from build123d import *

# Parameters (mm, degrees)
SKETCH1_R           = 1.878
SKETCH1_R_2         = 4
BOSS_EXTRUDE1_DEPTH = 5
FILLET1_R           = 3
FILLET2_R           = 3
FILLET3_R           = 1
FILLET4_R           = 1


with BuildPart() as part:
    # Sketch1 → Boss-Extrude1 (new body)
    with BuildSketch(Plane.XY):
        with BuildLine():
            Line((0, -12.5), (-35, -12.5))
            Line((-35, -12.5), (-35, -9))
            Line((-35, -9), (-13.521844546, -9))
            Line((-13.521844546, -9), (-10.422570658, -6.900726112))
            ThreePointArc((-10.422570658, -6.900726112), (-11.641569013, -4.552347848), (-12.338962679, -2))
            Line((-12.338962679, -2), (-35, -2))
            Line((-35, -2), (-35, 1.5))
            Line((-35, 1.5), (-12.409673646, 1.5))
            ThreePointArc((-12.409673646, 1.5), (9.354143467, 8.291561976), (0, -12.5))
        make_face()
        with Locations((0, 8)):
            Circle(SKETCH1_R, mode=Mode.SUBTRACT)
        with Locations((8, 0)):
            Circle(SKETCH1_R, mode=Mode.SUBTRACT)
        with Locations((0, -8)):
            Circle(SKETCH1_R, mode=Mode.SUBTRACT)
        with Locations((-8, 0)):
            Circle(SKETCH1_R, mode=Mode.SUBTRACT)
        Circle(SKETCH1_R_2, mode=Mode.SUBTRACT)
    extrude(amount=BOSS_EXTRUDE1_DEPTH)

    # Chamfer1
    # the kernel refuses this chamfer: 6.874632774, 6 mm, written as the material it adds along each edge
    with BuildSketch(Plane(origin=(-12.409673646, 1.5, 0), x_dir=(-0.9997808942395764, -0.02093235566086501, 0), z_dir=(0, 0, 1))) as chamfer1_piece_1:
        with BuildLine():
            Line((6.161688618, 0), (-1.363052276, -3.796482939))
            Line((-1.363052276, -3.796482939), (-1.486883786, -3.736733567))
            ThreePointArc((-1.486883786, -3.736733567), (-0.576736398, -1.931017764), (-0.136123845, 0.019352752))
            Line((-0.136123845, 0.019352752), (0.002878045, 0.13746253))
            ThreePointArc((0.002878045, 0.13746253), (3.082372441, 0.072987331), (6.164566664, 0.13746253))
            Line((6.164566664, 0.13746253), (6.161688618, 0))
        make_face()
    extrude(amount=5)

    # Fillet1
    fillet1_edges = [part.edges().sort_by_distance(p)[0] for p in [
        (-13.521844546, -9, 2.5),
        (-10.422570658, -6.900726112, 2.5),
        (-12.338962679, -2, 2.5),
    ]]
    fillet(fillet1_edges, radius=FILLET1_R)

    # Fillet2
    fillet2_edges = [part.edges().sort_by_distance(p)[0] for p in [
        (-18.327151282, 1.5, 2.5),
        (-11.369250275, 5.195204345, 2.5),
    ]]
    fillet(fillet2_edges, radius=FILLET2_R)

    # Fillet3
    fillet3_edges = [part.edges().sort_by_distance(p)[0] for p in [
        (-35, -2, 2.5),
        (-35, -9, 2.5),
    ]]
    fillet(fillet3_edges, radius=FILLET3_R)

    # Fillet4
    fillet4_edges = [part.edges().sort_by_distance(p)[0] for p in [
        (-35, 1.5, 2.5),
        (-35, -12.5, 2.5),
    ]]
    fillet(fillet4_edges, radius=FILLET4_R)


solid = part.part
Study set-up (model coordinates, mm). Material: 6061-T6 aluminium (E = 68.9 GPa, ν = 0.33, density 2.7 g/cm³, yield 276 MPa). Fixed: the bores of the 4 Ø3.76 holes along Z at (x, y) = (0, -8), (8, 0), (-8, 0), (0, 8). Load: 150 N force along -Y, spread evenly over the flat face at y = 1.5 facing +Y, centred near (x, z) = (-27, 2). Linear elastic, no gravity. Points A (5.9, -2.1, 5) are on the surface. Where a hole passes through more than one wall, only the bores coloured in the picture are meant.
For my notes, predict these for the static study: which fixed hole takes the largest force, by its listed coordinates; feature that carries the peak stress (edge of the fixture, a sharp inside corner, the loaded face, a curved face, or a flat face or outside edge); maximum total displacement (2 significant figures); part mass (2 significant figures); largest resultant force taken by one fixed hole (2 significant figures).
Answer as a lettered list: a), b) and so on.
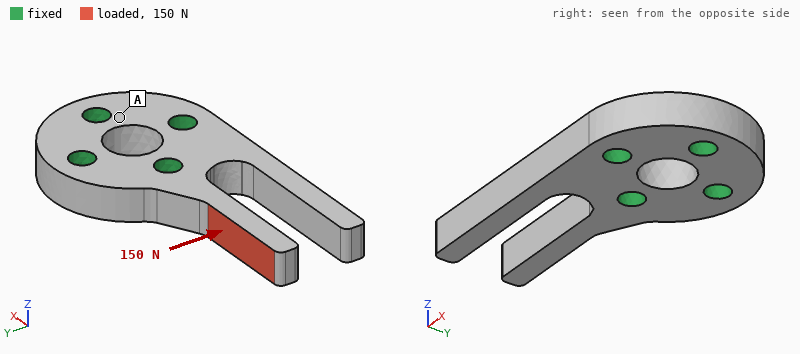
a) (0, 8)
b) a curved face
c) 0.15 mm
d) 8.0 g
e) 170 N
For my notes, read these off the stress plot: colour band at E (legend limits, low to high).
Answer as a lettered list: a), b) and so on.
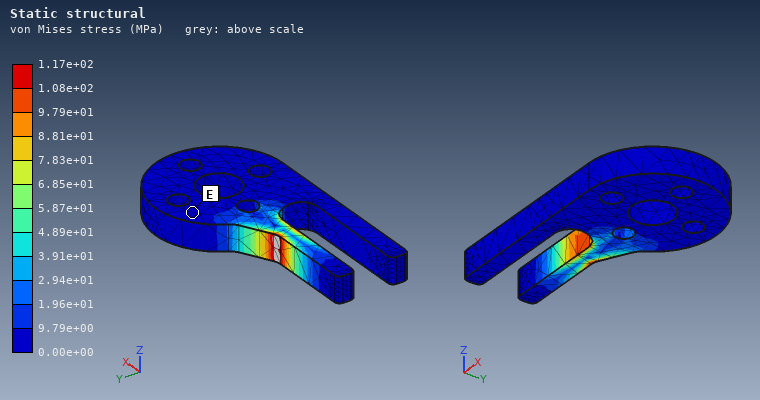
a) 0.00e+00 to 9.79e+00 MPa
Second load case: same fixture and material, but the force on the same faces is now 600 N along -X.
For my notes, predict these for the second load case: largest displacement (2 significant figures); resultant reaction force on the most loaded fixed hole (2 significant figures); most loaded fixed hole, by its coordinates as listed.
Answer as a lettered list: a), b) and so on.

a) 0.12 mm
b) 470 N
c) (-8, 0)
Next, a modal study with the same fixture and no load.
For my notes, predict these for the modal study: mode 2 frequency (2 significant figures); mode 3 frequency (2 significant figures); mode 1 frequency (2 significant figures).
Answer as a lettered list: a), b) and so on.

a) 5200 Hz
b) 7000 Hz
c) 4900 Hz
